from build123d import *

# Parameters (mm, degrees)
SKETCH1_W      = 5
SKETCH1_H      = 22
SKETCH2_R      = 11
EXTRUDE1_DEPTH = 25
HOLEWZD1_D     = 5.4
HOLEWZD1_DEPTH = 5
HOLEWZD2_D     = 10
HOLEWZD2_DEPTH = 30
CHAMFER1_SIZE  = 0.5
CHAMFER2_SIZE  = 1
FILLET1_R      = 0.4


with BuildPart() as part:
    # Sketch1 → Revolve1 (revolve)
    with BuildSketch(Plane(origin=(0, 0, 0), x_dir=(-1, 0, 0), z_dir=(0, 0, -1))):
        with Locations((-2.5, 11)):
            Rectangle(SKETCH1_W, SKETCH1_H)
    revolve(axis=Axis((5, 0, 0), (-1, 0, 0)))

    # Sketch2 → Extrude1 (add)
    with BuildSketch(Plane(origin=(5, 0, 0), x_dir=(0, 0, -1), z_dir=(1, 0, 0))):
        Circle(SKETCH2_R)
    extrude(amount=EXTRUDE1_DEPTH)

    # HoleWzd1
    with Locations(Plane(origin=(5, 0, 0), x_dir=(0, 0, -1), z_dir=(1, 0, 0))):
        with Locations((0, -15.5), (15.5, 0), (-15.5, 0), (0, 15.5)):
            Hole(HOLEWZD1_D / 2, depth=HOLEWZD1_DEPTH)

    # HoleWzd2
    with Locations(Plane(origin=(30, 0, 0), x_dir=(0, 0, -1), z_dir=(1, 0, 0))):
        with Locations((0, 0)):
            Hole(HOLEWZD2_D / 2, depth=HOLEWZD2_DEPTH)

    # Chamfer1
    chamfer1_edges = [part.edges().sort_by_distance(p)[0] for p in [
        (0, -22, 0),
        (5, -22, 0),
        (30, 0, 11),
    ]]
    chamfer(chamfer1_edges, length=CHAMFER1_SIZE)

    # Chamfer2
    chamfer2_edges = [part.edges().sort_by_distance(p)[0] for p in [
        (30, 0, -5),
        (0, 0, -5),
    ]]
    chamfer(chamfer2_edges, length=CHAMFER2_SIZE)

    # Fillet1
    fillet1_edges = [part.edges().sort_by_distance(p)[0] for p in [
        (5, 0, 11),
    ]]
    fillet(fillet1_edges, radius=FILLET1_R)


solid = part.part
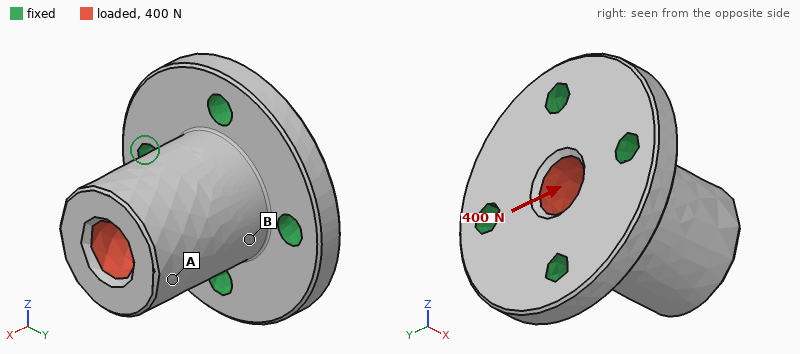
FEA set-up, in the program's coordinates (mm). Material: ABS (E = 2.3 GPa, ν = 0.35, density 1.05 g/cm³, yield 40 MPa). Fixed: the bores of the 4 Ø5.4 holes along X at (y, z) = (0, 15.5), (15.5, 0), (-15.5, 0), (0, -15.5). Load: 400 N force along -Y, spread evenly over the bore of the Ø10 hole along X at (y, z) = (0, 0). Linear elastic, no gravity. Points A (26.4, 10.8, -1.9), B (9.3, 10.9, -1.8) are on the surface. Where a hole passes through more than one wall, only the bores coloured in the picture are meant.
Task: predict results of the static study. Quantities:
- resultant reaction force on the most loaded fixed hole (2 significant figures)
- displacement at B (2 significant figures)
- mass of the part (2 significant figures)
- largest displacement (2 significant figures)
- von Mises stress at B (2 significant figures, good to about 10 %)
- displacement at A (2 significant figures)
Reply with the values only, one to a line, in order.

230 N
0.036 mm
15 g
0.11 mm
3.2 MPa
0.094 mm
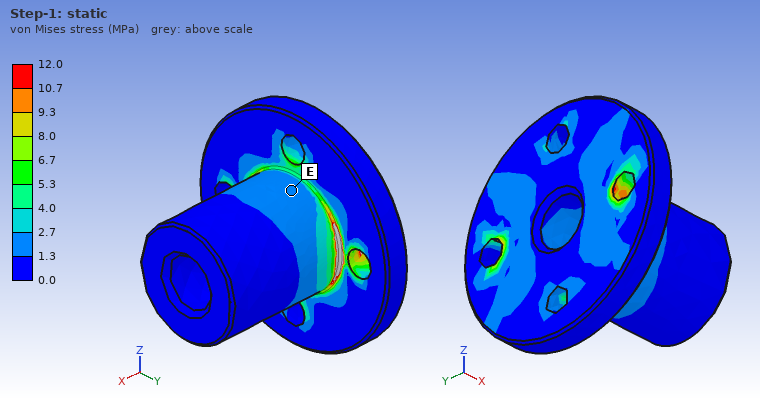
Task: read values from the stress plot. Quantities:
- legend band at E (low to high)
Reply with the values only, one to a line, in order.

1.3 to 2.7 MPa
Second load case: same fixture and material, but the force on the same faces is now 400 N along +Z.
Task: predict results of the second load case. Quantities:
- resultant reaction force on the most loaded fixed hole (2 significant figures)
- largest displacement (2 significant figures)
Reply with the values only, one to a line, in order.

230 N
0.11 mm
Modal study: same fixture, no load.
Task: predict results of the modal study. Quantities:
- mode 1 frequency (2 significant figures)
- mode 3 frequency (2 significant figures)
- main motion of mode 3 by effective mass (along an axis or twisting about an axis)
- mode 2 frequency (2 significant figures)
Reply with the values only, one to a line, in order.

3700 Hz
7700 Hz
along X
3700 Hz
